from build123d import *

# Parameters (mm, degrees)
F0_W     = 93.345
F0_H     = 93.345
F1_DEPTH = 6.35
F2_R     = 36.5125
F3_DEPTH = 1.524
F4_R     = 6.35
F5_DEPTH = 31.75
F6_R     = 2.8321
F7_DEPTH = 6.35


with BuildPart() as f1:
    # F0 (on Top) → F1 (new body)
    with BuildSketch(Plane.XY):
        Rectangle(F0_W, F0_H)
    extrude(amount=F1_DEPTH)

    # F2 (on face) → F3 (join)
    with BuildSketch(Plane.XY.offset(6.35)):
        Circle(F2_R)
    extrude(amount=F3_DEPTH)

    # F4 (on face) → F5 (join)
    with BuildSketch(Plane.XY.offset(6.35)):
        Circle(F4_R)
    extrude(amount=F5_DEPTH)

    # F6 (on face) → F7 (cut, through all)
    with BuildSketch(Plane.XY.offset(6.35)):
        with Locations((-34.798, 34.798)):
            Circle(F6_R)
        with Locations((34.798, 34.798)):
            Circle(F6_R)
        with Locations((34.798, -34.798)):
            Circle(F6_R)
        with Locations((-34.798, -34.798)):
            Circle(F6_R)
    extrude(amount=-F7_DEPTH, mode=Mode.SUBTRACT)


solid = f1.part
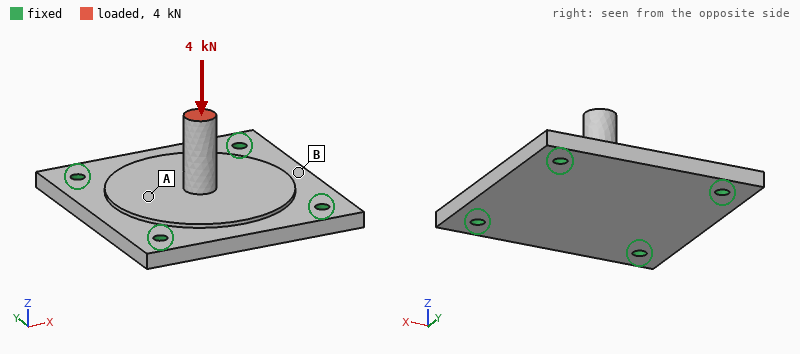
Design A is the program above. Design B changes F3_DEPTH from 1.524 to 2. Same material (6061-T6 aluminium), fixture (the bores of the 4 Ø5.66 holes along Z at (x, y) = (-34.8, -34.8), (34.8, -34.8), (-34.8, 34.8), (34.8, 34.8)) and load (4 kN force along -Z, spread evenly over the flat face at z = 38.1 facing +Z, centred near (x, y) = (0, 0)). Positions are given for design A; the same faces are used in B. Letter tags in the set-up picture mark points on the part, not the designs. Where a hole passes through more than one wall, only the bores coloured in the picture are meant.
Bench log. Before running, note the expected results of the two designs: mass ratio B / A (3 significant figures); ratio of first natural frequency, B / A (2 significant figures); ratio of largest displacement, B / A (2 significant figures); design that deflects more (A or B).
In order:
1.03
1.0
0.90
A
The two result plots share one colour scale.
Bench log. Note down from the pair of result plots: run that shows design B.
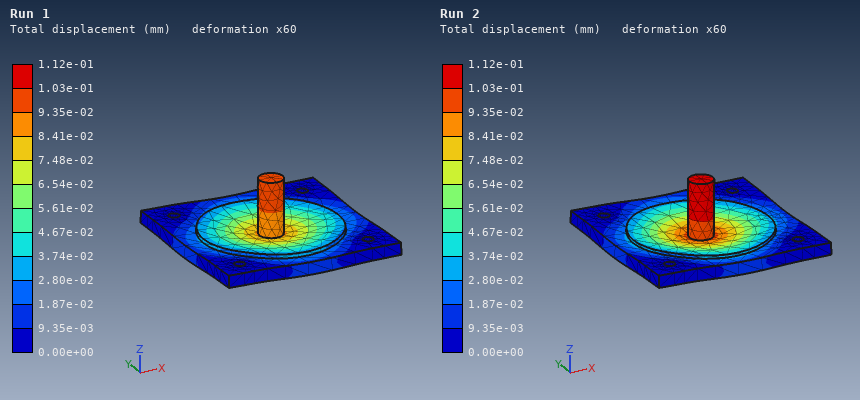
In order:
Run 1
